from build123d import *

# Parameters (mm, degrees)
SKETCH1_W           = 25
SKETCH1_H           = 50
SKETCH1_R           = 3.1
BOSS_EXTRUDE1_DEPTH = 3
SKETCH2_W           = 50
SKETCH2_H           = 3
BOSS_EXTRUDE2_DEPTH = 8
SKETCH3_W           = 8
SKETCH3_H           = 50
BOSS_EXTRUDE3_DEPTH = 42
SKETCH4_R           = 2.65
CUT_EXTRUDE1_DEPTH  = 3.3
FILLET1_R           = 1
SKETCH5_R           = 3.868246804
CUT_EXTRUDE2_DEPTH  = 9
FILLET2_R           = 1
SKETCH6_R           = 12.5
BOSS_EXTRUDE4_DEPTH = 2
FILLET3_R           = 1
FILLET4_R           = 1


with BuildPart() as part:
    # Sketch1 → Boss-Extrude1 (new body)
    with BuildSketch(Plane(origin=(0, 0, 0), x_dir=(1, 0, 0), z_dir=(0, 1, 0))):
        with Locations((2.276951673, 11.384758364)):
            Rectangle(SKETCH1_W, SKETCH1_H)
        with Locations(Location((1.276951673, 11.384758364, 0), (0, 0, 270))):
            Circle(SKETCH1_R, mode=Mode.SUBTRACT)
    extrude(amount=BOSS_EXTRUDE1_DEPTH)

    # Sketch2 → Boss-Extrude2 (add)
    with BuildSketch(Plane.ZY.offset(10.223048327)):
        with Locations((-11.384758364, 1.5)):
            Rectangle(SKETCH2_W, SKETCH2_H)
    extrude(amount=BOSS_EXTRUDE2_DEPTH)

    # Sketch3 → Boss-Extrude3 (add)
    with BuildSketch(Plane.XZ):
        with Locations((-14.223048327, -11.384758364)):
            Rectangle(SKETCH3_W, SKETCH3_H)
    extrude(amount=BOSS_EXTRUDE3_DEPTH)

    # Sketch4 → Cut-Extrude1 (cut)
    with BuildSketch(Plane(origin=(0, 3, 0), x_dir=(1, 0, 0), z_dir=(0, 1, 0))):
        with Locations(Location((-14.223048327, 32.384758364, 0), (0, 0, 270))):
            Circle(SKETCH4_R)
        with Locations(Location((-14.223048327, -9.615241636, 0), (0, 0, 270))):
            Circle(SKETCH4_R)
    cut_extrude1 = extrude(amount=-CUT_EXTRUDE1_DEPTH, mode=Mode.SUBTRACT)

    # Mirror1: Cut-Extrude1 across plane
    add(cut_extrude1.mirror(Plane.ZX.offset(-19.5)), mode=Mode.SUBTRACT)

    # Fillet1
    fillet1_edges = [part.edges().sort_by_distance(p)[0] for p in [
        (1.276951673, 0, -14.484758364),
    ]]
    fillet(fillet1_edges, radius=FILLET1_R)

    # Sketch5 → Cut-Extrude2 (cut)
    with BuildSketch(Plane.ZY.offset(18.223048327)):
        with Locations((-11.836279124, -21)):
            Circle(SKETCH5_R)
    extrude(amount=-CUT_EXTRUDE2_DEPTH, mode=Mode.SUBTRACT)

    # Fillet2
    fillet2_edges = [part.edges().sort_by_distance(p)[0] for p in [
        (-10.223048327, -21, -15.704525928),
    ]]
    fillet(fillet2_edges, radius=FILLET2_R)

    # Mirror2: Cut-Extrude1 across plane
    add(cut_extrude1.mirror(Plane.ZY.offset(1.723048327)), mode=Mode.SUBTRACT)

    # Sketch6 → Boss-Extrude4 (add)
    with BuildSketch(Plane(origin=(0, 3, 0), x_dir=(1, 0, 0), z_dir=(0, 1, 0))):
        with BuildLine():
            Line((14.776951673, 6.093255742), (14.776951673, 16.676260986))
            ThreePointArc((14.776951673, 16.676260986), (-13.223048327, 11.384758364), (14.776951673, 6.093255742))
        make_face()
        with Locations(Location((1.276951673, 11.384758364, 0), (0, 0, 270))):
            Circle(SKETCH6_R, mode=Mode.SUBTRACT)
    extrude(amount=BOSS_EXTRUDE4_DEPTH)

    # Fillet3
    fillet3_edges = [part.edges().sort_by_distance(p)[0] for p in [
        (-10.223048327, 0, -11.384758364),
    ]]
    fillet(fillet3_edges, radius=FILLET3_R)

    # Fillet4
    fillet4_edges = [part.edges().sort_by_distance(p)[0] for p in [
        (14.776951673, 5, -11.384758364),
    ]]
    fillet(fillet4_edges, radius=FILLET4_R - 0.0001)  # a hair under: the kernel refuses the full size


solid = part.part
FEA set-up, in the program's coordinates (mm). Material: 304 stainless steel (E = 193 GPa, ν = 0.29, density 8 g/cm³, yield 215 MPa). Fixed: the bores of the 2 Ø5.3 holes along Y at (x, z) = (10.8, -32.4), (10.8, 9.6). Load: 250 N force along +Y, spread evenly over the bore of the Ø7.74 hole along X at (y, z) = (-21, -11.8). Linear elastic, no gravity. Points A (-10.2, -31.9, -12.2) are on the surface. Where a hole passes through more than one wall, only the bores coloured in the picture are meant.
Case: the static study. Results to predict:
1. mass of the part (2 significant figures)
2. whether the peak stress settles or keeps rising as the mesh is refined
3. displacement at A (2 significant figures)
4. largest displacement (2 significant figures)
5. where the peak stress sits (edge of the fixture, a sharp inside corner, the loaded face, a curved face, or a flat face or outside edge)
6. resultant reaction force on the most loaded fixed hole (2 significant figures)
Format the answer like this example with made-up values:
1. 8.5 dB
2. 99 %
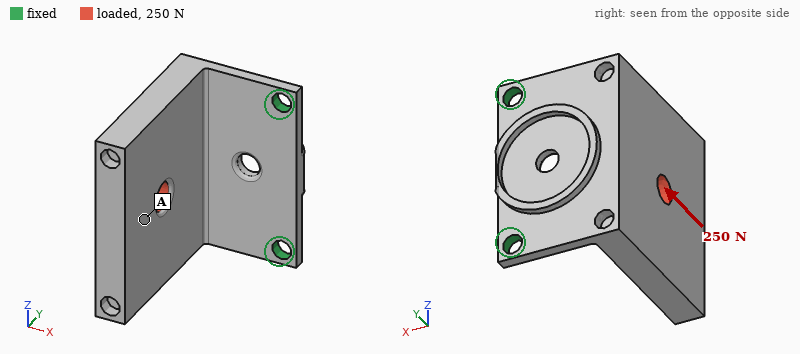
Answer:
1. 170 g
2. keeps rising
3. 0.13 mm
4. 0.17 mm
5. edge of the fixture
6. 130 N
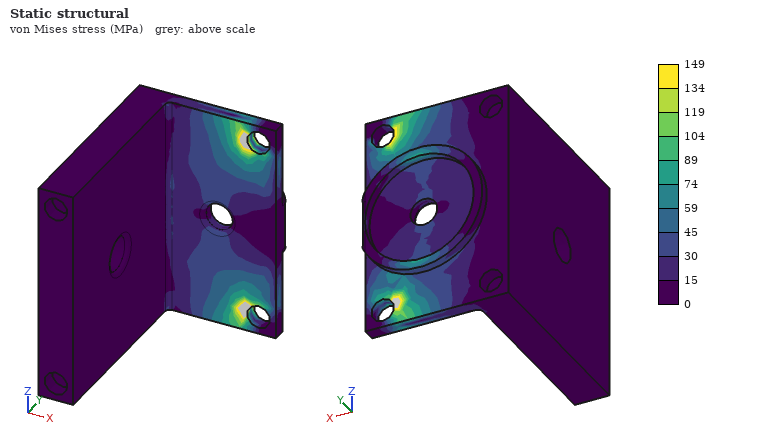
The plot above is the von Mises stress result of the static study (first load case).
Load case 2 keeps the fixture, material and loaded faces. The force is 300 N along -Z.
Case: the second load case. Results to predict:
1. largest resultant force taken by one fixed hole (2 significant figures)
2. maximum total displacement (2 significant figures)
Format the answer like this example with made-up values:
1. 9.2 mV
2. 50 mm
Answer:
1. 280 N
2. 48 µm
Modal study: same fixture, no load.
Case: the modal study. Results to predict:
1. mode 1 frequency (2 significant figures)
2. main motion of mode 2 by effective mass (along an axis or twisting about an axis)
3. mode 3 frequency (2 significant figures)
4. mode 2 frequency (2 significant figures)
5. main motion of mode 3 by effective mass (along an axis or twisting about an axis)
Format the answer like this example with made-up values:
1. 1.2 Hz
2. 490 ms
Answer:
1. 480 Hz
2. along Z
3. 2100 Hz
4. 1300 Hz
5. along Y
